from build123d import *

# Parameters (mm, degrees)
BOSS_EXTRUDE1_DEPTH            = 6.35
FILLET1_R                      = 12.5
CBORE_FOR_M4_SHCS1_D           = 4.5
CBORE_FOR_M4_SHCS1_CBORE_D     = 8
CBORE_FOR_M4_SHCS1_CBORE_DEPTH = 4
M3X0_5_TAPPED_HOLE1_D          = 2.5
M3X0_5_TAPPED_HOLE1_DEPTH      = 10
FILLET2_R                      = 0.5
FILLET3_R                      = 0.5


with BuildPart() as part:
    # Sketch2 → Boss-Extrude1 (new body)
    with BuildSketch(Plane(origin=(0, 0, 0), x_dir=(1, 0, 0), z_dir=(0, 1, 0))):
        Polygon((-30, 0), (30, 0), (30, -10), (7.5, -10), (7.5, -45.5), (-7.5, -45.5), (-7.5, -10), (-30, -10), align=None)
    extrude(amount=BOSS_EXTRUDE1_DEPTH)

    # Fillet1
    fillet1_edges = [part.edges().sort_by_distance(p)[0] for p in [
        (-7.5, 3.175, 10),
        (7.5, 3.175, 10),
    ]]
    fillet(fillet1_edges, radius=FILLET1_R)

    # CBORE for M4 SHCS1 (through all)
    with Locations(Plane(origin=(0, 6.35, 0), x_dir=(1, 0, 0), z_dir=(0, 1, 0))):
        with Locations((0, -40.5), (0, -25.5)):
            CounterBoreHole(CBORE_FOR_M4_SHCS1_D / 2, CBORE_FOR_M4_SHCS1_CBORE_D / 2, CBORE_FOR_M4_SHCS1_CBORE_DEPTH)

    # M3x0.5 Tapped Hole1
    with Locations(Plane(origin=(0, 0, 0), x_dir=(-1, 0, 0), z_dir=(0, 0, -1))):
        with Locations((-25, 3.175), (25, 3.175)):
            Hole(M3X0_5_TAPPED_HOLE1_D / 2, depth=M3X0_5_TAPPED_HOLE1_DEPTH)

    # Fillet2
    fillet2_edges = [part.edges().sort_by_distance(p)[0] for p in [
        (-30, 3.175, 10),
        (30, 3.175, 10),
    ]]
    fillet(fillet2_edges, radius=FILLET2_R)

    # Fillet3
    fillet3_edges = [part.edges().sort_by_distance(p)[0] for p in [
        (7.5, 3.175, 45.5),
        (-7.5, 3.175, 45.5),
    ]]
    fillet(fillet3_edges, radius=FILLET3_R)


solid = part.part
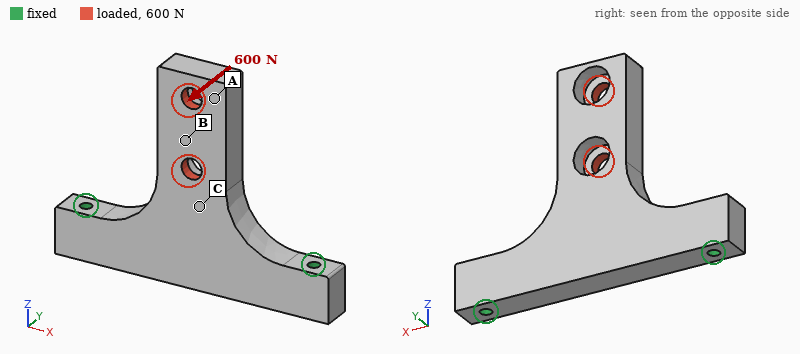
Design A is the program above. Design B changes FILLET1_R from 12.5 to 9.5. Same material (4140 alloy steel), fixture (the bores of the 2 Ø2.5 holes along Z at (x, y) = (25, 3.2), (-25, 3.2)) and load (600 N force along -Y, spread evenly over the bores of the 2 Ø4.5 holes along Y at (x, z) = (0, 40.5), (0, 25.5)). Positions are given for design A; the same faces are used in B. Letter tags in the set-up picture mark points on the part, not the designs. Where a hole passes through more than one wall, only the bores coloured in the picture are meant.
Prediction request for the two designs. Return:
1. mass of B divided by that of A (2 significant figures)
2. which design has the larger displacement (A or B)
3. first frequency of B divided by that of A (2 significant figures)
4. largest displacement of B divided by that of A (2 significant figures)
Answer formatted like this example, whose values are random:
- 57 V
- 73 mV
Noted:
- 0.97
- B
- 0.95
- 1.1
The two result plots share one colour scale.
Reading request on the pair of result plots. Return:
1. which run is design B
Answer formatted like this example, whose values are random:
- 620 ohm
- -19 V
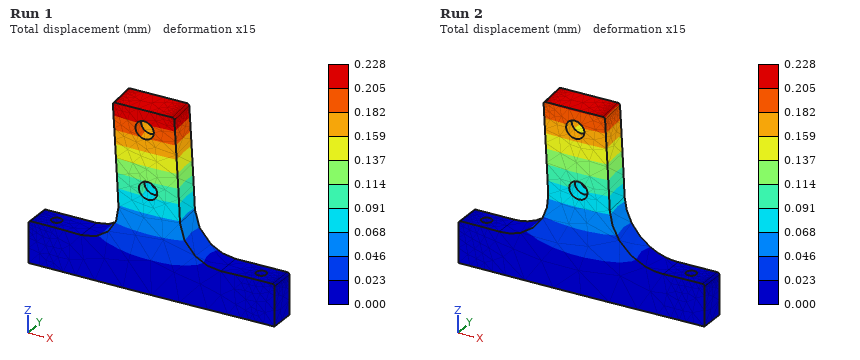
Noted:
- Run 1
